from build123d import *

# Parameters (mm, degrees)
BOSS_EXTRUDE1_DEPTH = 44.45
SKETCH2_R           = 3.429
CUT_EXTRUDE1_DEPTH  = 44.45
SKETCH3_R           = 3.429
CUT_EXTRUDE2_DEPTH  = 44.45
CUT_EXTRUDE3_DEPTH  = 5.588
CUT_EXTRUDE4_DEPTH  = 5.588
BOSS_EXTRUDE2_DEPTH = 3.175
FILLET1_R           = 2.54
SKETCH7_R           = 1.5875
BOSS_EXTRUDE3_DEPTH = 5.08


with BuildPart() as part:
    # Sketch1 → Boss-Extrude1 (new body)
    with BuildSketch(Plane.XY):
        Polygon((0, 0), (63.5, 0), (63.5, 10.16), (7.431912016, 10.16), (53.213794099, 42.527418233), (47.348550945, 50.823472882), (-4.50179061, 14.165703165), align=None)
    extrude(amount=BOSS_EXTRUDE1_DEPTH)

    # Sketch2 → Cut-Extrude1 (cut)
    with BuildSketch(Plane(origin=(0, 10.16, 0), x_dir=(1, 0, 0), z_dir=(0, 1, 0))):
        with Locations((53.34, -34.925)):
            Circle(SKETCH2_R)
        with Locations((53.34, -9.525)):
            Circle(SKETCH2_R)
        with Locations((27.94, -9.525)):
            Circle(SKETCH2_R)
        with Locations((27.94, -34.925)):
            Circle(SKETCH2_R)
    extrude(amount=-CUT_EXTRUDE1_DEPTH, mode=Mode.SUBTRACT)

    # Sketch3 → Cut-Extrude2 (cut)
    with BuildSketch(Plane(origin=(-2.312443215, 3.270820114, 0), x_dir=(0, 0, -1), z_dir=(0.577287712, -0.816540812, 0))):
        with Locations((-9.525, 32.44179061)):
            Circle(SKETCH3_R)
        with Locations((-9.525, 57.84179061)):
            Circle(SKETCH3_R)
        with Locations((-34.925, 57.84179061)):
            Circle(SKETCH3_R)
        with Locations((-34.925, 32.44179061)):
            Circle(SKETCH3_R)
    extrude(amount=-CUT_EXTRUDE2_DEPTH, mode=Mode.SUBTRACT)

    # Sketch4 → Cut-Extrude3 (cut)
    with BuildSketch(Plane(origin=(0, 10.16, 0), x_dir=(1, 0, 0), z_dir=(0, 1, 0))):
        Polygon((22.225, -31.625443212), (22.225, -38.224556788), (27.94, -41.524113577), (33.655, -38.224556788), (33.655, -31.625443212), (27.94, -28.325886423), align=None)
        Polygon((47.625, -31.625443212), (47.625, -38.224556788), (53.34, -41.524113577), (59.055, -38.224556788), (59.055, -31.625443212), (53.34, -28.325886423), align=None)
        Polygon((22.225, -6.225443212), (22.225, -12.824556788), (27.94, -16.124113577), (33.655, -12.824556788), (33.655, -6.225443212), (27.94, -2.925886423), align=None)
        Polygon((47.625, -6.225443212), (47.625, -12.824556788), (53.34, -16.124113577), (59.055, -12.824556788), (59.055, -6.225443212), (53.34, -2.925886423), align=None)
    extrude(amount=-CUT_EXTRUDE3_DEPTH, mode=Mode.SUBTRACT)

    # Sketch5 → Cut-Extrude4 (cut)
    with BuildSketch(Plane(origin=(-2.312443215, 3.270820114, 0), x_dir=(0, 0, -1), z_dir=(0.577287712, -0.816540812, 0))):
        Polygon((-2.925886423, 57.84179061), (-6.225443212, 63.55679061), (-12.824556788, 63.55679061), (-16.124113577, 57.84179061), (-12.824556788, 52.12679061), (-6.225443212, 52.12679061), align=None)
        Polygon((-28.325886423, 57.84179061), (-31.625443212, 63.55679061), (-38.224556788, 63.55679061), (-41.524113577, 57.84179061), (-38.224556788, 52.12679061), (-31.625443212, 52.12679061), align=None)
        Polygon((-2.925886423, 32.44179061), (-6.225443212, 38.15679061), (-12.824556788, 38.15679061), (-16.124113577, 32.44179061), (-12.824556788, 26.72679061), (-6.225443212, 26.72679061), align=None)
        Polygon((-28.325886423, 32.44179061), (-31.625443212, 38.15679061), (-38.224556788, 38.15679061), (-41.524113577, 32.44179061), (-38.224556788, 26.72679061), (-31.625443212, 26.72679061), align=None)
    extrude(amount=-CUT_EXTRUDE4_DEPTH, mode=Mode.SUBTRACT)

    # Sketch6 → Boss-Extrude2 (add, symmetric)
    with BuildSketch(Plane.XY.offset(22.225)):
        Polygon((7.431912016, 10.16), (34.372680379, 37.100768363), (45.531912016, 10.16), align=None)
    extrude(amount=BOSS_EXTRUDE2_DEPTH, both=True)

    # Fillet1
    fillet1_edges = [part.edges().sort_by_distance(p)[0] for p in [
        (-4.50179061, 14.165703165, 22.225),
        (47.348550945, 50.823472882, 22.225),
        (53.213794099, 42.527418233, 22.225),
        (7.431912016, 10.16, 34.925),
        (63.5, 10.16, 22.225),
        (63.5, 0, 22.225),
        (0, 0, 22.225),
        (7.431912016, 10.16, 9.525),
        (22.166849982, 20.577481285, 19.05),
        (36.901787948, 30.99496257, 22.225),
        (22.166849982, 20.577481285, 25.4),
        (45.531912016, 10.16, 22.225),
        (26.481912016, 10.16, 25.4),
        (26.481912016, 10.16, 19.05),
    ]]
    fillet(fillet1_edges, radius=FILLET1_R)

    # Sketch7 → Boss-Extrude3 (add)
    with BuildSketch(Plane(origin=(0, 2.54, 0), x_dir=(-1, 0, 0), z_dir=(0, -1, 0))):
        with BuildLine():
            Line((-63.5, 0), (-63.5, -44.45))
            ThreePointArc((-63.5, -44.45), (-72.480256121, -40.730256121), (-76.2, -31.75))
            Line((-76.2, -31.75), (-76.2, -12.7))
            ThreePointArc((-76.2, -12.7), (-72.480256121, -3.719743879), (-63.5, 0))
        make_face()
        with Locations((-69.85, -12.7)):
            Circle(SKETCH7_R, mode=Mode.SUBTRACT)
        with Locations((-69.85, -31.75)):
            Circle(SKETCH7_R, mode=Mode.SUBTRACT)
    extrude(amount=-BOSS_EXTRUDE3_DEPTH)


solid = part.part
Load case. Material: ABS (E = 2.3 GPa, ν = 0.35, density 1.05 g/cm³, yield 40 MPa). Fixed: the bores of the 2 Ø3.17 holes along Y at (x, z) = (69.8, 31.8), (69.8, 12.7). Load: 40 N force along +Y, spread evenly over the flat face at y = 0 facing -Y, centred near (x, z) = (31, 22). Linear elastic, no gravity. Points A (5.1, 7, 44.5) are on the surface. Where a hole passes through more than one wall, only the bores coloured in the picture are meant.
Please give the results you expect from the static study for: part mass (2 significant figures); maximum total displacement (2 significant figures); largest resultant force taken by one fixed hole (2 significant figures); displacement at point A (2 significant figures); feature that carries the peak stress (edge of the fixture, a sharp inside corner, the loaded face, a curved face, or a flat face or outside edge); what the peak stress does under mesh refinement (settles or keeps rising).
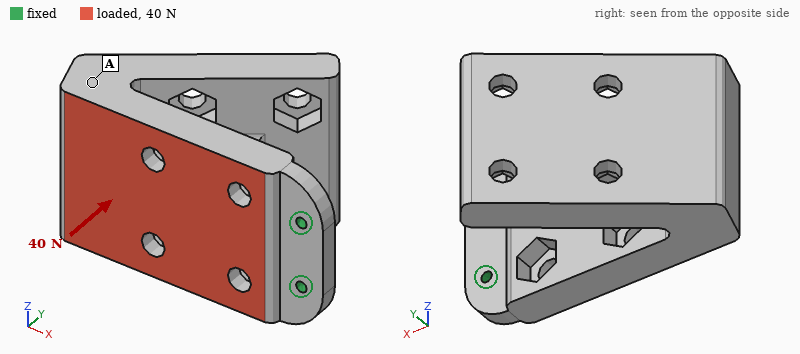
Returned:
59 g
1.1 mm
20 N
0.91 mm
edge of the fixture
keeps rising
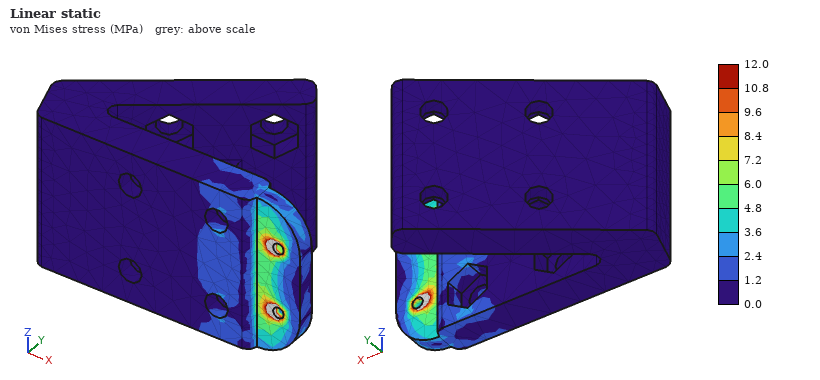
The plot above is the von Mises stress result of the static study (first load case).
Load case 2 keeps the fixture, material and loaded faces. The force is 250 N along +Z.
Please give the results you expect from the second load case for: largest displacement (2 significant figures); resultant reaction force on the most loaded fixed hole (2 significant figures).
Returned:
0.41 mm
480 N
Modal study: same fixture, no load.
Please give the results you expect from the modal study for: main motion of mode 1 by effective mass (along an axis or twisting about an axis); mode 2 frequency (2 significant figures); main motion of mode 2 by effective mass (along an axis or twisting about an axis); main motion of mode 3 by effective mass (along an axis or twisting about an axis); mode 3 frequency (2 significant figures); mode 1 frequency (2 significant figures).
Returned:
along Y
370 Hz
along Z
along Z
710 Hz
140 Hz
